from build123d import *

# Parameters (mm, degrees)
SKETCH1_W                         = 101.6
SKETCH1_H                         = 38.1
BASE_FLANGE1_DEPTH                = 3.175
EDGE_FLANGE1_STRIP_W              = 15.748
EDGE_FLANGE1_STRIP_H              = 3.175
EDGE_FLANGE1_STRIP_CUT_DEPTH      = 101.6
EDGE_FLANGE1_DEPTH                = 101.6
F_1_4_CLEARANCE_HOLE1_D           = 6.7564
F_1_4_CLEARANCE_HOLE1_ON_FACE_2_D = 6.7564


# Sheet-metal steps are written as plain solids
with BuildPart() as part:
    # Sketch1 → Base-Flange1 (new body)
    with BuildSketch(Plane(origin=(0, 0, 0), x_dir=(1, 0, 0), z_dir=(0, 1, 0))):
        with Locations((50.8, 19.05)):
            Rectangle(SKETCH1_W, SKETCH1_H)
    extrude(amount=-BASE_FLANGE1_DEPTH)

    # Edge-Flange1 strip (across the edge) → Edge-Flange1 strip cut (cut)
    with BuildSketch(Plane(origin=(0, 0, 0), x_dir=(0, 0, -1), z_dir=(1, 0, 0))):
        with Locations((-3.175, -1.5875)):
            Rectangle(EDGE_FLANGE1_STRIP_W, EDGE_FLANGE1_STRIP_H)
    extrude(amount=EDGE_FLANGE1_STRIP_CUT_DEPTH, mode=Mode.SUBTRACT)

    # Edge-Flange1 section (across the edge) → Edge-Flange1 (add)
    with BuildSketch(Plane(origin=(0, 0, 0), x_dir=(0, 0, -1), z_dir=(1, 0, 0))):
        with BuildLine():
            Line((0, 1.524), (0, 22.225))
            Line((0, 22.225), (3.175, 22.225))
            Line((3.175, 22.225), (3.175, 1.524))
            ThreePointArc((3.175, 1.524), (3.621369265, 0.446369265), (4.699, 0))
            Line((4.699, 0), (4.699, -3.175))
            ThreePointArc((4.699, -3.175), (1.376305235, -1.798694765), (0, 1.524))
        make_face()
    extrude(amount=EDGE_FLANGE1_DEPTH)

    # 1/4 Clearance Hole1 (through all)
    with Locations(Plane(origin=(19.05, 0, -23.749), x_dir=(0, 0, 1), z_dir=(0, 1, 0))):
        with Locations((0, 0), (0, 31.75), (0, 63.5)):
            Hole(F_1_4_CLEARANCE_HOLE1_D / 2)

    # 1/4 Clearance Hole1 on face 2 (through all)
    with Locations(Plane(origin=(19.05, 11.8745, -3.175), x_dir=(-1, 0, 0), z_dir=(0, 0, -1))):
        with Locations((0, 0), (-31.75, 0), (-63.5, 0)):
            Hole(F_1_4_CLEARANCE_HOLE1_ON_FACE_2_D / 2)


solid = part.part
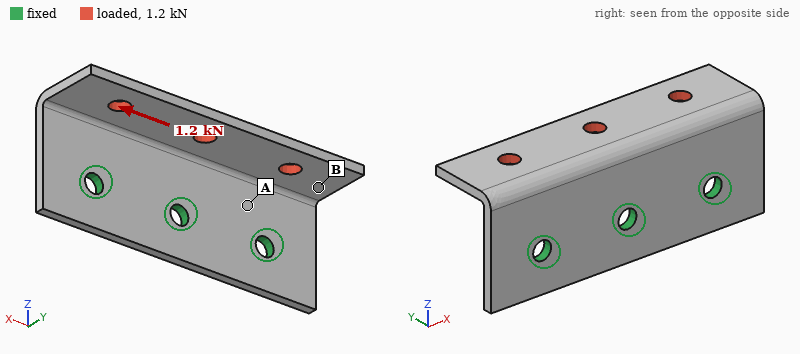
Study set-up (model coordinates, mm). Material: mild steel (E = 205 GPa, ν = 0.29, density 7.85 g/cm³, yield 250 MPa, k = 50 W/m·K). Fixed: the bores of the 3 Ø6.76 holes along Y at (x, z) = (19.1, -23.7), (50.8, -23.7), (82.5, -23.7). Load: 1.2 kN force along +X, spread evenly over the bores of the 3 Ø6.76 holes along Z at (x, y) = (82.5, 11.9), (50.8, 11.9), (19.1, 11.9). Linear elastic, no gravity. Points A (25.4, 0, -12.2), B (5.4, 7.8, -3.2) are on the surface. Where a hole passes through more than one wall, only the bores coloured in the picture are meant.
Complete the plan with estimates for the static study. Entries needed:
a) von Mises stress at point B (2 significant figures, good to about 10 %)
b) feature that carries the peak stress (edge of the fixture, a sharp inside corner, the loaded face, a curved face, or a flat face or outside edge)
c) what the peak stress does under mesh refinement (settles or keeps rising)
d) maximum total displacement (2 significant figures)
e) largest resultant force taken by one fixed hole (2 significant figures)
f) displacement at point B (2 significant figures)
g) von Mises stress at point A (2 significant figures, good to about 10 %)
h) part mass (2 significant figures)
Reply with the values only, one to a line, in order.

13 MPa
edge of the fixture
keeps rising
57 µm
570 N
36 µm
35 MPa
140 g
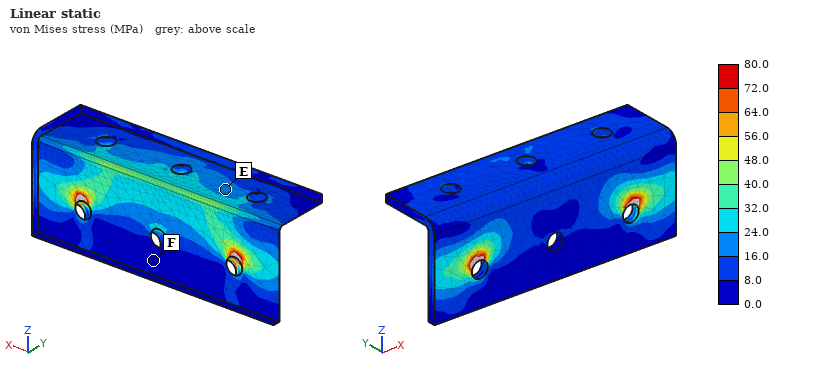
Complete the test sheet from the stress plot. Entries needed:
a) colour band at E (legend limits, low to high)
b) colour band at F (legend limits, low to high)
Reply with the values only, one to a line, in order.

16.0 to 24.0 MPa
0.0 to 8.0 MPa
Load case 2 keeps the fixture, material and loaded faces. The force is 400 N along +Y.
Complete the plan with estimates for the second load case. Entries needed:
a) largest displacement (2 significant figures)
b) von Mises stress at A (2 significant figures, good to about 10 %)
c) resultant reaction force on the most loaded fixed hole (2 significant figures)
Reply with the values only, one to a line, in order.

47 µm
24 MPa
130 N
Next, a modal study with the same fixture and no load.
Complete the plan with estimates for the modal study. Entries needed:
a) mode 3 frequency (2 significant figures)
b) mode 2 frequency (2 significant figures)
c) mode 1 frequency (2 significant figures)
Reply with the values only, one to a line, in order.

4800 Hz
2300 Hz
1800 Hz
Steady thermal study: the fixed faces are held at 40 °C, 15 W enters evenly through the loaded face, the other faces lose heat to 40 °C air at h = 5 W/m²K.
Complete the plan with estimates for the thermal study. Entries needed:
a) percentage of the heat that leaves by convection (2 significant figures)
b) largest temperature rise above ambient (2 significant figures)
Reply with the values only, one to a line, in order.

6.8 %
39 K
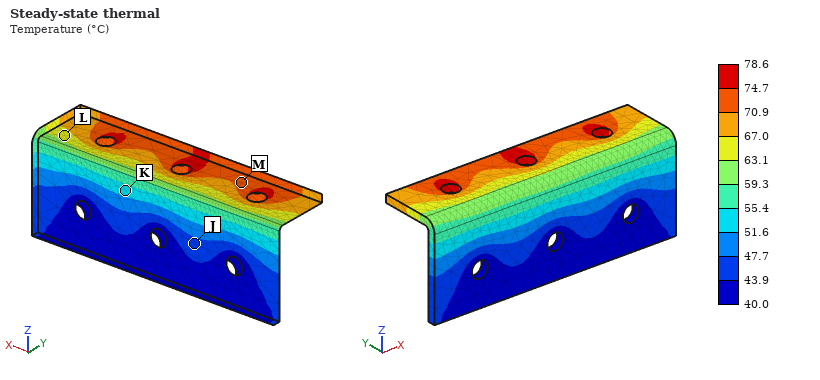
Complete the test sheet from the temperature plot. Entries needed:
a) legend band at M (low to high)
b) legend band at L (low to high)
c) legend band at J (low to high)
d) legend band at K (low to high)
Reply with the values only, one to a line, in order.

70.9 to 74.7 °C
63.1 to 67.0 °C
43.9 to 47.7 °C
51.6 to 55.4 °C
